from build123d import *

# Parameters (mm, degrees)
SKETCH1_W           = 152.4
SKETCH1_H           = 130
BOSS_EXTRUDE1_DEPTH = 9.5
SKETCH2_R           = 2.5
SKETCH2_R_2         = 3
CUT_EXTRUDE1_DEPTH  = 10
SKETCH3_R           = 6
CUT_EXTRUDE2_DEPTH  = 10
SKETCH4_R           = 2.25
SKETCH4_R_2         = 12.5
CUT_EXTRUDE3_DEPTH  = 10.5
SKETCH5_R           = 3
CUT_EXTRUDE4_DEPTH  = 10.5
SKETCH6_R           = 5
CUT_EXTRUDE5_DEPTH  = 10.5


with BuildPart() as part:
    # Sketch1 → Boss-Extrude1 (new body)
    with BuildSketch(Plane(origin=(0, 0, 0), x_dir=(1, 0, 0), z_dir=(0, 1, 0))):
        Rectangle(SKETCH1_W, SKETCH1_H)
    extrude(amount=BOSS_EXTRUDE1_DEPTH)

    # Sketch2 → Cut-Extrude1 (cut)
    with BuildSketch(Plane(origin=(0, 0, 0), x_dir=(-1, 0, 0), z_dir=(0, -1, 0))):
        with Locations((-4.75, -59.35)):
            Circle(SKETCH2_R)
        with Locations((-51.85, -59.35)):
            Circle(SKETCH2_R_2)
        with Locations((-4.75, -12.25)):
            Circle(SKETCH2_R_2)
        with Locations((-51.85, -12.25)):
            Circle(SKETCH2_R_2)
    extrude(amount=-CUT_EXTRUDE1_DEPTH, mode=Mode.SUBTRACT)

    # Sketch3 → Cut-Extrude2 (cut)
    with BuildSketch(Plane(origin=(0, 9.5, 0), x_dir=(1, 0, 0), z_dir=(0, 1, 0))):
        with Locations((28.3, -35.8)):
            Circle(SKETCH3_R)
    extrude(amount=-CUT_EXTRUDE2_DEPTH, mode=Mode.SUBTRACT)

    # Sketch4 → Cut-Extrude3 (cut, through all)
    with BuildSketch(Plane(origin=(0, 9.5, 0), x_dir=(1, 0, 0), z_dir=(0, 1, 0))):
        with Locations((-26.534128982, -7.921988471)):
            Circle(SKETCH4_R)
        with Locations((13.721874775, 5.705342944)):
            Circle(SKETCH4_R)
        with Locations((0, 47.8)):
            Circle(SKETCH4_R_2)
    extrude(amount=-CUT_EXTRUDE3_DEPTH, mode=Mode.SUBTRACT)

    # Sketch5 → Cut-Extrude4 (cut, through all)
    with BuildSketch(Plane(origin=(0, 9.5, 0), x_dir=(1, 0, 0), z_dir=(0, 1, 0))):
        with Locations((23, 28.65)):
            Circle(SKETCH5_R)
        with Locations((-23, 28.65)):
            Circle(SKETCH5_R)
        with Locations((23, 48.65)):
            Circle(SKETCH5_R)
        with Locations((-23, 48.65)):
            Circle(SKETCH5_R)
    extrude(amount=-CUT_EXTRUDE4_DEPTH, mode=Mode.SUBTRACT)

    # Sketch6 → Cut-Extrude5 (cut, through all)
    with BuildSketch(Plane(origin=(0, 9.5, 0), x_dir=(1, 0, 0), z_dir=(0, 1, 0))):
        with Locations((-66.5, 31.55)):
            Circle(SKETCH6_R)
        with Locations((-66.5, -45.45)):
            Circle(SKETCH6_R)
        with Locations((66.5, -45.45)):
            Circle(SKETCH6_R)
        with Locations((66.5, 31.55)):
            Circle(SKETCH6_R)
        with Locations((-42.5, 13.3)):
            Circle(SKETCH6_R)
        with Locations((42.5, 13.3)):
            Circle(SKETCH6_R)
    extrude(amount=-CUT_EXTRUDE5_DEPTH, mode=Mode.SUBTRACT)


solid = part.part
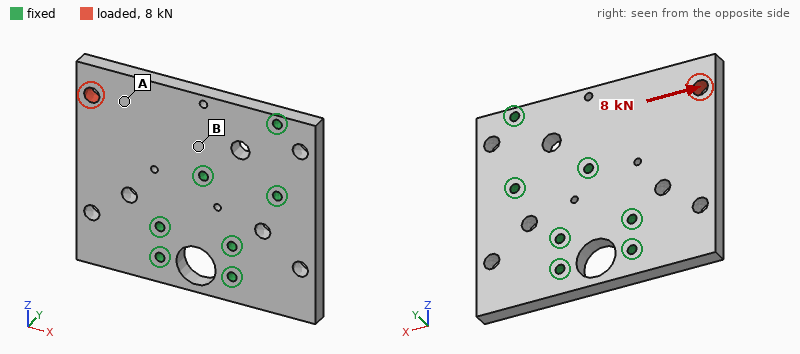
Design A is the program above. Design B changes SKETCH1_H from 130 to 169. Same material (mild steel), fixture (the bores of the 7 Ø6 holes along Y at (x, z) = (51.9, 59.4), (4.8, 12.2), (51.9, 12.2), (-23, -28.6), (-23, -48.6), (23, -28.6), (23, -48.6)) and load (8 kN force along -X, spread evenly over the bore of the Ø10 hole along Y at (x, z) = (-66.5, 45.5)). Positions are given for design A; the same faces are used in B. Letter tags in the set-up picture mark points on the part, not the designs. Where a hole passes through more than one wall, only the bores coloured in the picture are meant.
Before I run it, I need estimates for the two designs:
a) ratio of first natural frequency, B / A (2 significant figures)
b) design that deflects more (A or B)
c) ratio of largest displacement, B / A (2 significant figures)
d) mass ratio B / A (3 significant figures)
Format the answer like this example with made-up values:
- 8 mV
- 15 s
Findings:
- 0.79
- A
- 0.78
- 1.32
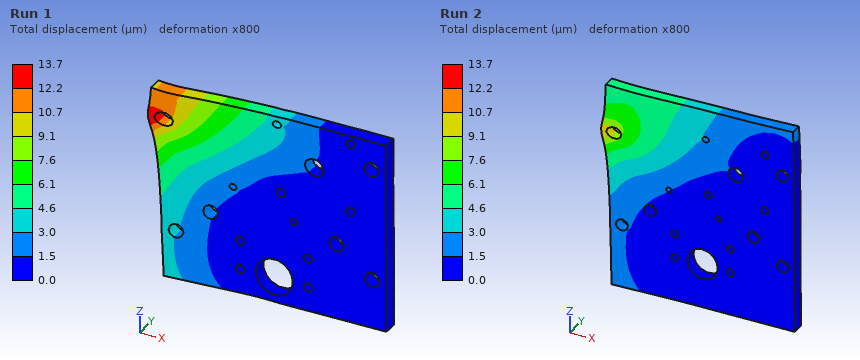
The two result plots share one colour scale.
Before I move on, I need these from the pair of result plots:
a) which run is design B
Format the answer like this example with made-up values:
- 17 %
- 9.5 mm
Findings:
- Run 2
